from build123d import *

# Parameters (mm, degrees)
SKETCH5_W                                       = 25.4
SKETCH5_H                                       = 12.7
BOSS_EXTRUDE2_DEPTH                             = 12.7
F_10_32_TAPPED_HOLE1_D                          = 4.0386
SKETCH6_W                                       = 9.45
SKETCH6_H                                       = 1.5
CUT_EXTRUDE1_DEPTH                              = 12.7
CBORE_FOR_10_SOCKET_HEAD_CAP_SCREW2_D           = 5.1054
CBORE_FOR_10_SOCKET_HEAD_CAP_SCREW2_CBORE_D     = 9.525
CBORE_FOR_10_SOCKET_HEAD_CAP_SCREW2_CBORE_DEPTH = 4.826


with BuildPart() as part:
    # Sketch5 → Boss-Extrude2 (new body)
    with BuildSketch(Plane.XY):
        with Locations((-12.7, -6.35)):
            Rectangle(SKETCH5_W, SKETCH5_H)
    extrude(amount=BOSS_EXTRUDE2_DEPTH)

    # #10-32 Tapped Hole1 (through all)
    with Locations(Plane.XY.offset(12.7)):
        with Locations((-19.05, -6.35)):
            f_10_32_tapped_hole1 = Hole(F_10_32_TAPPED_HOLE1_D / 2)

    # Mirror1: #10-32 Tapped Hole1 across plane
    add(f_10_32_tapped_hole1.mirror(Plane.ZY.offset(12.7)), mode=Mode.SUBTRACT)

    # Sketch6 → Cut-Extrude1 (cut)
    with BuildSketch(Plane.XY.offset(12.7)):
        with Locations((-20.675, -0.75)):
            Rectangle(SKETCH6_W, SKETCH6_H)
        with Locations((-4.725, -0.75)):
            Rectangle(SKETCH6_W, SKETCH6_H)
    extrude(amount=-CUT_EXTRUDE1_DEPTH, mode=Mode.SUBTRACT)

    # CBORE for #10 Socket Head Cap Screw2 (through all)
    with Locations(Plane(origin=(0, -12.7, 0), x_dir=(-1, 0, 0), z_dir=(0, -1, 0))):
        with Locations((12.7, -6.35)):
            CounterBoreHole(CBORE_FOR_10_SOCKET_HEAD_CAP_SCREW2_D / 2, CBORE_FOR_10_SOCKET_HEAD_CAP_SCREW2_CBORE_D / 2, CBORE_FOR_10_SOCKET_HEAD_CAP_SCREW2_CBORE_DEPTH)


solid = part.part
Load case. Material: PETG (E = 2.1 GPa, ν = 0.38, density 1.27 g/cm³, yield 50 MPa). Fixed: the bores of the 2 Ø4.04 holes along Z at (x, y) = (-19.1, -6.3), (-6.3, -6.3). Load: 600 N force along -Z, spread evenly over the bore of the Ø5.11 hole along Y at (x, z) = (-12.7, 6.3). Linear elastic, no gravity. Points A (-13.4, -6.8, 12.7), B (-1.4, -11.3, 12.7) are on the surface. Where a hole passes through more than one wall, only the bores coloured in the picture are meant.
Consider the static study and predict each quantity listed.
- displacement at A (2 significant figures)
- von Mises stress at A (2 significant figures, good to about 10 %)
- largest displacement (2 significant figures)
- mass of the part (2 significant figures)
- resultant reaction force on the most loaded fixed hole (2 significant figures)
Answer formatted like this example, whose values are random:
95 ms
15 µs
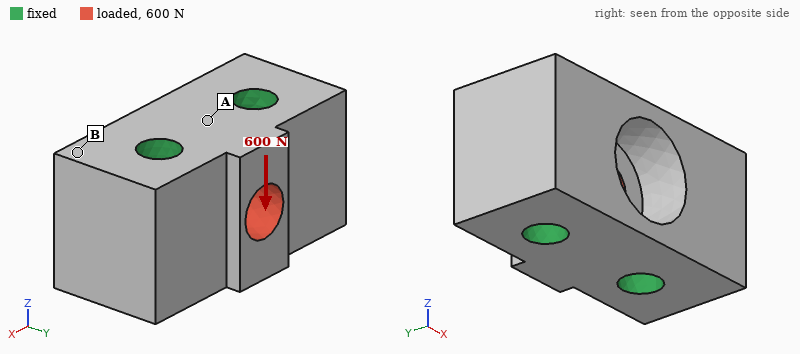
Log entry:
14 µm
3.6 MPa
38 µm
3.7 g
300 N
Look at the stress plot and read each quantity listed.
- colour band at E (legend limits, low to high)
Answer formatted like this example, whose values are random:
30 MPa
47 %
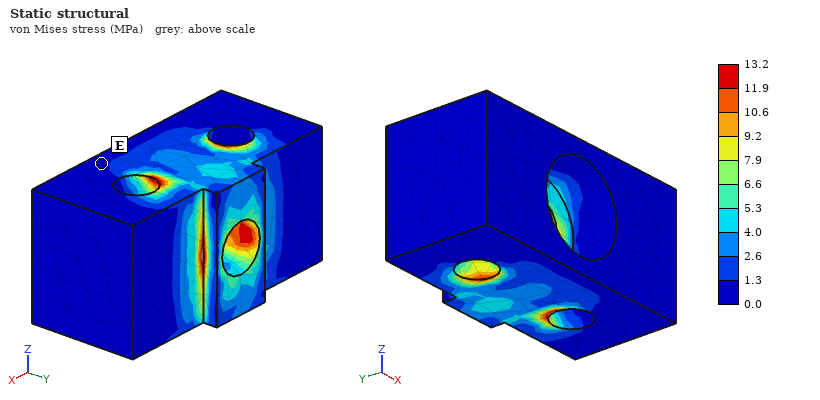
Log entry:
0.0 to 1.3 MPa
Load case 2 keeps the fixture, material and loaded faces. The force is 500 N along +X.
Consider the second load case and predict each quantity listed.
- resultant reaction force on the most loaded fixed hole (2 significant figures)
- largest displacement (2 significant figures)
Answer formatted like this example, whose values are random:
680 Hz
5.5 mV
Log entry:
260 N
41 µm
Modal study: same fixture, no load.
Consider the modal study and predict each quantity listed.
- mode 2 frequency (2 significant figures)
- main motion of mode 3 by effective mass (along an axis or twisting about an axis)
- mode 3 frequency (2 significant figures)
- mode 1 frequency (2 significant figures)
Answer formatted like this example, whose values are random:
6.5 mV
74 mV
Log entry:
20 kHz
along Z
26 kHz
20 kHz
